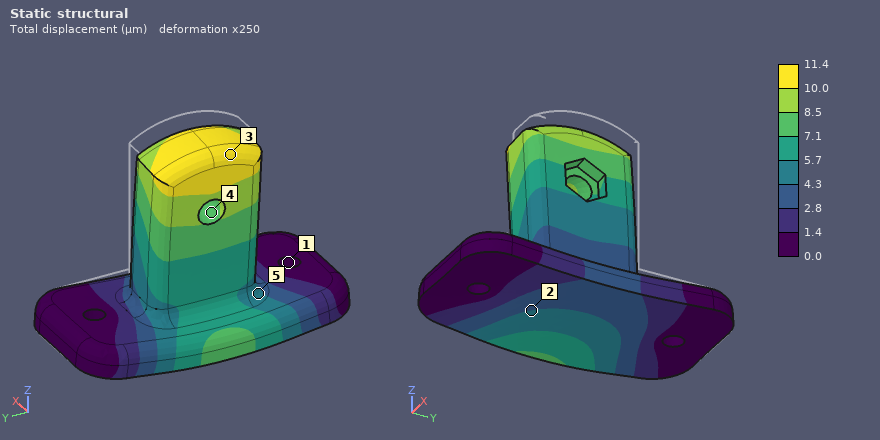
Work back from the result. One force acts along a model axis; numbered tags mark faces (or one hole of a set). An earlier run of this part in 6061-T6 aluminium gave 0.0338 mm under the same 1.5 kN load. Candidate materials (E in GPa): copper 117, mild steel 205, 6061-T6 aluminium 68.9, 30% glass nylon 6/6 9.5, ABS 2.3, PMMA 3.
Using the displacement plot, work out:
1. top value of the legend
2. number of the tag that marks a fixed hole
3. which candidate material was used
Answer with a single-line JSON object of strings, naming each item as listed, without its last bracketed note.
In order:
{"top value of the legend": "11.4 µm", "number of the tag that marks a fixed hole": "1", "which candidate material was used": "mild steel"}
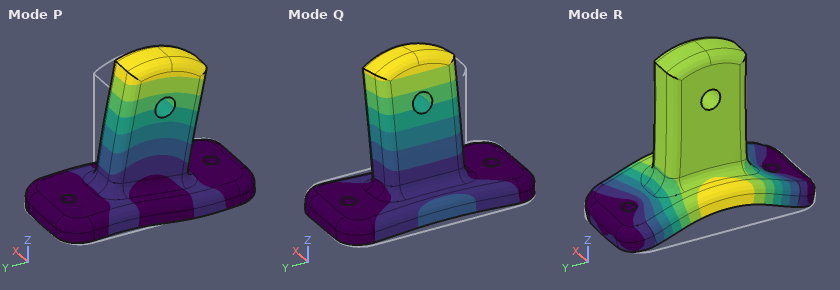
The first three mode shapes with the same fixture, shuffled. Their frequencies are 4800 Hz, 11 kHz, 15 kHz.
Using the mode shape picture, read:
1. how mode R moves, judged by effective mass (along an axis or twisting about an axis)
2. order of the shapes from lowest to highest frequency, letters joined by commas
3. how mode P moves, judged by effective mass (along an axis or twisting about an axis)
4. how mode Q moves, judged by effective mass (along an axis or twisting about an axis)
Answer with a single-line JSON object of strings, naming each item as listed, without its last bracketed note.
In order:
{"how mode R moves, judged by effective mass": "along Z", "order of the shapes from lowest to highest frequency, letters joined by commas": "Q, P, R", "how mode P moves, judged by effective mass": "along Y", "how mode Q moves, judged by effective mass": "along X"}
